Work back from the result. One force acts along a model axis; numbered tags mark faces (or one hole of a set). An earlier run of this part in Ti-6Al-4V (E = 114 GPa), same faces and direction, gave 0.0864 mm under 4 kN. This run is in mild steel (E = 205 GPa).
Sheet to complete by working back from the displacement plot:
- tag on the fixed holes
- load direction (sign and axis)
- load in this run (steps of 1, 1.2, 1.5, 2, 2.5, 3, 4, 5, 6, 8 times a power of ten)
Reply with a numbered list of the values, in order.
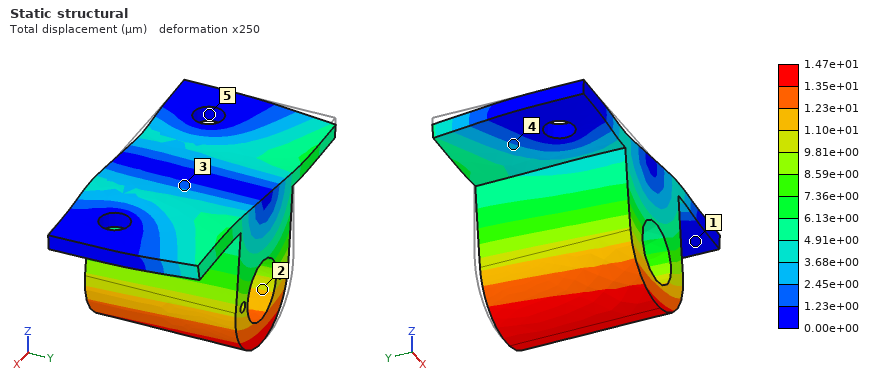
1. 5
2. +X
3. 1.2 kN
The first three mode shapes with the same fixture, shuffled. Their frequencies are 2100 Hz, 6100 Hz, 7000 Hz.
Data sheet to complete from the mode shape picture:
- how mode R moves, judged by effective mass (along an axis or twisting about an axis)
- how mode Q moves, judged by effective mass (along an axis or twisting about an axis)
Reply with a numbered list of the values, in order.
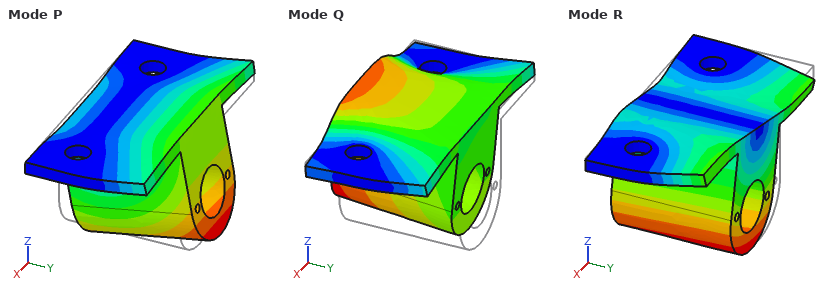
1. along X
2. along Z
